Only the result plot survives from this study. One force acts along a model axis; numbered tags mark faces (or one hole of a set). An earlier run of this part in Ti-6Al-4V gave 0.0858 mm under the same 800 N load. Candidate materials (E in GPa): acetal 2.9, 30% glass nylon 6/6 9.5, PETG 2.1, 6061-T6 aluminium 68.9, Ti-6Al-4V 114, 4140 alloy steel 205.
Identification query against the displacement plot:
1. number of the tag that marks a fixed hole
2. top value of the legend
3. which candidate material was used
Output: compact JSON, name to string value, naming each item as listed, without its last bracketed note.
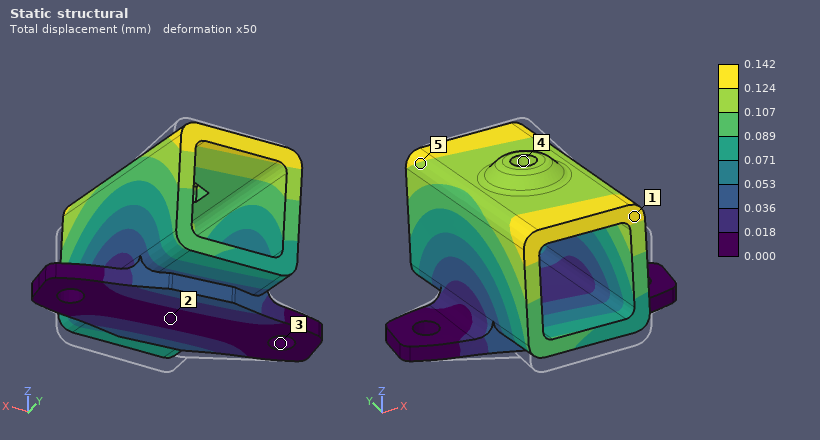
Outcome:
{"number of the tag that marks a fixed hole": "3", "top value of the legend": "0.142 mm", "which candidate material was used": "6061-T6 aluminium"}
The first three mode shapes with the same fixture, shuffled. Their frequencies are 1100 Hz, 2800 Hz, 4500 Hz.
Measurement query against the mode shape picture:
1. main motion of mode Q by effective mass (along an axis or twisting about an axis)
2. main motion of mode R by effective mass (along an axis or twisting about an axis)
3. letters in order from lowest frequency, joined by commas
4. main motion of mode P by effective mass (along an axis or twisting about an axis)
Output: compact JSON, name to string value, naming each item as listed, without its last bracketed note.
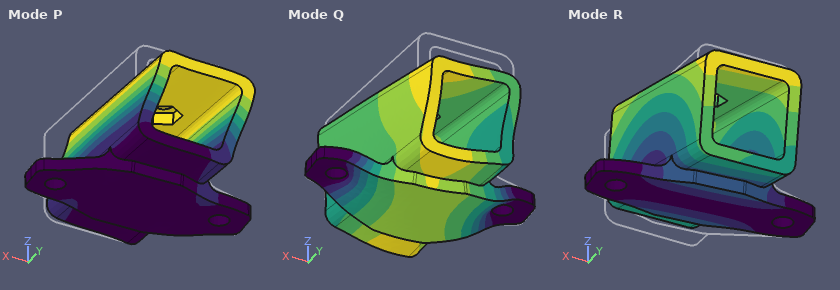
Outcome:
{"main motion of mode Q by effective mass": "along Z", "main motion of mode R by effective mass": "along Y", "letters in order from lowest frequency, joined by commas": "R, P, Q", "main motion of mode P by effective mass": "along X"}
